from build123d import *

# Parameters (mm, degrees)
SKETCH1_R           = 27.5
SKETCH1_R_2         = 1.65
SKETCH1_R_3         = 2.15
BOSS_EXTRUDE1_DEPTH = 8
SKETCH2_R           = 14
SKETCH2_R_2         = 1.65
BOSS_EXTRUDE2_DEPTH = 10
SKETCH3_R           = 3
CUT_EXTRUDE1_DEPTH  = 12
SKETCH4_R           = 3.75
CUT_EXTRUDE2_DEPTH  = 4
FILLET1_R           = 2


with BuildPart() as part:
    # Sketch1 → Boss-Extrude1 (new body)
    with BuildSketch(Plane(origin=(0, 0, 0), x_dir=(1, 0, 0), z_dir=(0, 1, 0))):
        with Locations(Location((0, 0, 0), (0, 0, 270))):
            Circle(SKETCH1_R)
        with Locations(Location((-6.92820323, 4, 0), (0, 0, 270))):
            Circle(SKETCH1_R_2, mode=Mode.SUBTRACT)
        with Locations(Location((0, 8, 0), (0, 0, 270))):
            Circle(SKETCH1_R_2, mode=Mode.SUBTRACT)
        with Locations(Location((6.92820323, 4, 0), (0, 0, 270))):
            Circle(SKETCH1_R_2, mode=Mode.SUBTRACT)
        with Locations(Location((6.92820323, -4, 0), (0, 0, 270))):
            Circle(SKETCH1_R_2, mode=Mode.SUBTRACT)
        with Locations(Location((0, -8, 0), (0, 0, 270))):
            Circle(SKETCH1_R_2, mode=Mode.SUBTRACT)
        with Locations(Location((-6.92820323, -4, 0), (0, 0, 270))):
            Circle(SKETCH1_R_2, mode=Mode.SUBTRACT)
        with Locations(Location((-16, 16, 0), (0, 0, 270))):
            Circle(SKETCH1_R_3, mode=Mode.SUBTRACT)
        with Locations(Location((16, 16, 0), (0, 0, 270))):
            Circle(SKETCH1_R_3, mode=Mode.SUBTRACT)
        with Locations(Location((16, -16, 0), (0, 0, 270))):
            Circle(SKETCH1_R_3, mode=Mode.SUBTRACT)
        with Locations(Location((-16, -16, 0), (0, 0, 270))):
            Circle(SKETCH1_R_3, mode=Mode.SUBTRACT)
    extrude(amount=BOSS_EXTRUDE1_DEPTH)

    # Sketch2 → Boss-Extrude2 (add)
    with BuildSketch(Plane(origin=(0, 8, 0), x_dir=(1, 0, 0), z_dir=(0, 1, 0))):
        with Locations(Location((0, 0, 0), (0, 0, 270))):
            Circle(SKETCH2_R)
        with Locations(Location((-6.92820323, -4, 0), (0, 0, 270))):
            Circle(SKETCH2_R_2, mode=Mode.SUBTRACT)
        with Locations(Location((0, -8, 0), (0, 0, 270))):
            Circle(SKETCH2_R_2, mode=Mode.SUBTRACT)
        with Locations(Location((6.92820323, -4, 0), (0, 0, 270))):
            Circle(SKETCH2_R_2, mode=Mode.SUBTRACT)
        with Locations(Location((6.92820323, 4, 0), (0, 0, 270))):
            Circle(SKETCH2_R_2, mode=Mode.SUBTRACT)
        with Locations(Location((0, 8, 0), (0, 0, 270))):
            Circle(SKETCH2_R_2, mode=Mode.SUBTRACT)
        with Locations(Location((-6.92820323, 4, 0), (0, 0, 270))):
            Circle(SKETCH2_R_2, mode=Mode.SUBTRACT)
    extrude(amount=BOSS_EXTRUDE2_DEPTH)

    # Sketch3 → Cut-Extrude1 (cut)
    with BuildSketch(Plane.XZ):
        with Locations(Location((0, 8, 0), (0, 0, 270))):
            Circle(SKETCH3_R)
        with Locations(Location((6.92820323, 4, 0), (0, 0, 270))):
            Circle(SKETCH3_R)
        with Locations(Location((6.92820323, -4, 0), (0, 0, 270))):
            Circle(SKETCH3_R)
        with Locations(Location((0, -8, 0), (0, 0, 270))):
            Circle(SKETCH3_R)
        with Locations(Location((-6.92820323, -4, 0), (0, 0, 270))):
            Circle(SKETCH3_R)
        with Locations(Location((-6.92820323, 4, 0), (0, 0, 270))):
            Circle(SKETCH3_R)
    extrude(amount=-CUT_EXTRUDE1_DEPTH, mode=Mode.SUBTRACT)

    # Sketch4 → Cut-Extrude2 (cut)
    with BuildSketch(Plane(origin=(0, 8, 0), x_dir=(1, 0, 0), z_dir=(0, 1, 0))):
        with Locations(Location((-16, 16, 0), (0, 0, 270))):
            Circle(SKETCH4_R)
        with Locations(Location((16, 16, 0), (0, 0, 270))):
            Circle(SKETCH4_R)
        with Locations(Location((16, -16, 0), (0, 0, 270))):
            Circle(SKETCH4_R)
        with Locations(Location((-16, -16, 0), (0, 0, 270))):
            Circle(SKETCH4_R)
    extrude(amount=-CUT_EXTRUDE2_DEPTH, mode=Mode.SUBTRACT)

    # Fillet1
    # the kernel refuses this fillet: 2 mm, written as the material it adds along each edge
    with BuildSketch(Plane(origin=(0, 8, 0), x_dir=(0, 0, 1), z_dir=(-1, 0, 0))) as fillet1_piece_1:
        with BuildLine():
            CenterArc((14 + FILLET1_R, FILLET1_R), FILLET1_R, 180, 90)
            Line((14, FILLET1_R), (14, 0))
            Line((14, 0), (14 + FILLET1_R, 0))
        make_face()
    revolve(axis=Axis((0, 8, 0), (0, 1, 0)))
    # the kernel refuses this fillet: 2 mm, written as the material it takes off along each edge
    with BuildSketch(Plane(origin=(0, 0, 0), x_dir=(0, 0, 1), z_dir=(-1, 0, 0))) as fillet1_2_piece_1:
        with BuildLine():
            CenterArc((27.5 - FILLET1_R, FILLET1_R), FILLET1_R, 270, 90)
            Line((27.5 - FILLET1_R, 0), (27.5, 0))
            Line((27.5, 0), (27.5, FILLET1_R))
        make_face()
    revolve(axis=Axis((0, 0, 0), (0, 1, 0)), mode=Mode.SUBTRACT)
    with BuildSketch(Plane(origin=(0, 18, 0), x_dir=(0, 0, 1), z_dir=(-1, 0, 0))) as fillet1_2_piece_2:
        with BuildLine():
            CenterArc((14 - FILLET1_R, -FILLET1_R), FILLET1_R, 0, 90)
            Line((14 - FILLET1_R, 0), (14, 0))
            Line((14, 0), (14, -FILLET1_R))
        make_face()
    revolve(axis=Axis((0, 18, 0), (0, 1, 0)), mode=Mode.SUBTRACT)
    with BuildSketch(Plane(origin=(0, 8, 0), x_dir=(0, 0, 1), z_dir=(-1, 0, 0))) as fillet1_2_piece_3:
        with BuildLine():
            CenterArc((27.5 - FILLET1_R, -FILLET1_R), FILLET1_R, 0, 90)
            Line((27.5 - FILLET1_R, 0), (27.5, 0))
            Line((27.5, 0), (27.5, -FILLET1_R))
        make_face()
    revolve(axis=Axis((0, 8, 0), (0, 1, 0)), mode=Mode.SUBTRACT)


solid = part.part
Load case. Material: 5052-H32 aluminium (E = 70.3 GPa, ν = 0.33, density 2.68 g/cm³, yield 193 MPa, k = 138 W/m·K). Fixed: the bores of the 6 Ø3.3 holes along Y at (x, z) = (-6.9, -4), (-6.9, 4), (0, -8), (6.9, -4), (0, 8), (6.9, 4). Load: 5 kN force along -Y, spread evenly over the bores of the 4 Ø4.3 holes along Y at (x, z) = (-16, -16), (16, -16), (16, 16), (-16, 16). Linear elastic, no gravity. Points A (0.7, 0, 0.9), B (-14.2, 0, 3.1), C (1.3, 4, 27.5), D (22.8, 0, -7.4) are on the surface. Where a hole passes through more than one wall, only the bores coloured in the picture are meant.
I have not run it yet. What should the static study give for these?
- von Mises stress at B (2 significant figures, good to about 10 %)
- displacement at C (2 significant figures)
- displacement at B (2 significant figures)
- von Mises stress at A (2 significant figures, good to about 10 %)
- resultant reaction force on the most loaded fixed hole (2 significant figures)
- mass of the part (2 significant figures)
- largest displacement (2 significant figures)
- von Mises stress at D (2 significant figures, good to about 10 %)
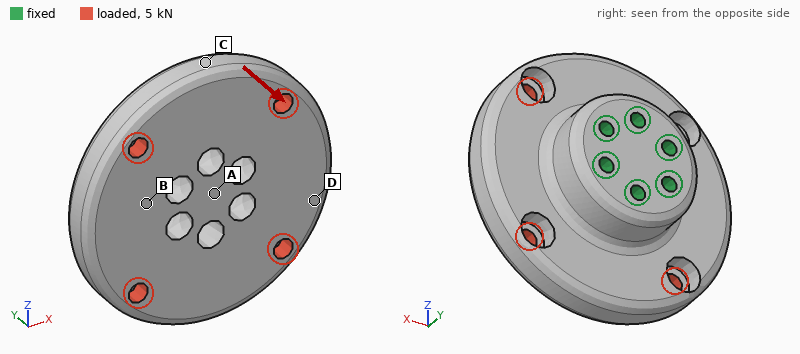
28 MPa
11 µm
5.6 µm
14 MPa
890 N
58 g
24 µm
24 MPa
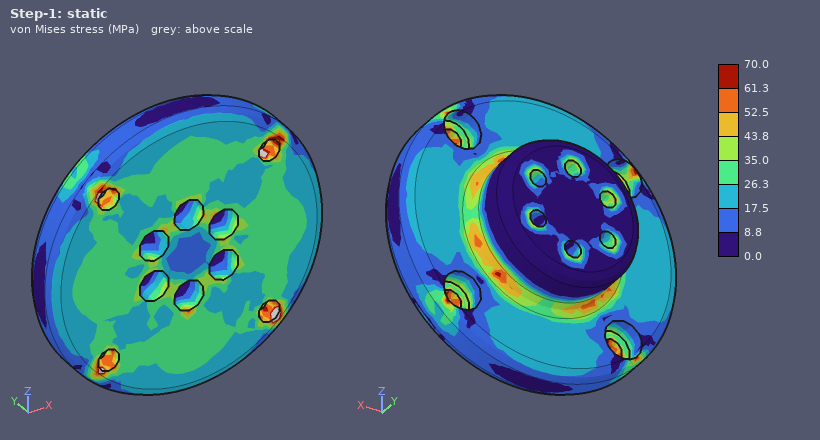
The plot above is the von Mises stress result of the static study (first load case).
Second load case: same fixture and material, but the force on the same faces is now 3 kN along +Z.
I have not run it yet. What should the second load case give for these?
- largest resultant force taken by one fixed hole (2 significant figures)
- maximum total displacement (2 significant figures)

1.2 kN
16 µm
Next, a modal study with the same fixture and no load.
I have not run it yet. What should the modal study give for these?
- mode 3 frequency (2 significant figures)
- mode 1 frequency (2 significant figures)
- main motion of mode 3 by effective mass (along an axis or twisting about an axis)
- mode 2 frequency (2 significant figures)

13 kHz
11 kHz
twisting about Y
11 kHz
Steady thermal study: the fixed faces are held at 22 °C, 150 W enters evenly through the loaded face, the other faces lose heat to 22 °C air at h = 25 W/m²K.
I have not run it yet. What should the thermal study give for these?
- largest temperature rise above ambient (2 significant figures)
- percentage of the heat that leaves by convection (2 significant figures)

56 K
3.6 %
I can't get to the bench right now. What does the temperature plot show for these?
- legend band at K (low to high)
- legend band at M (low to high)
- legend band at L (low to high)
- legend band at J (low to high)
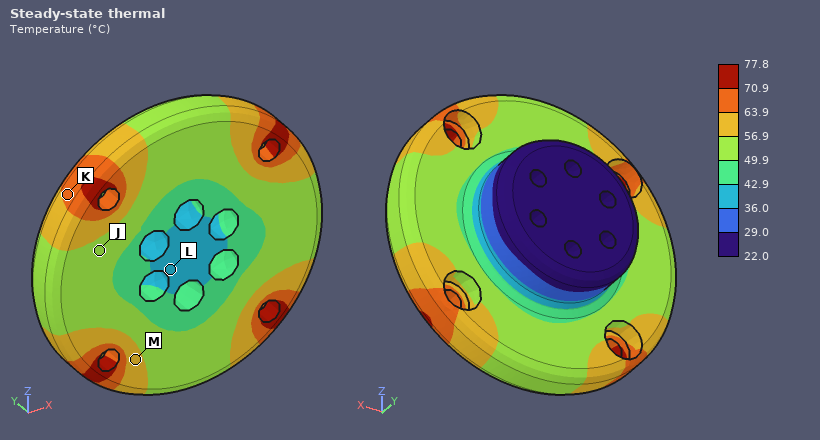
63.9 to 70.9 °C
56.9 to 63.9 °C
36.0 to 42.9 °C
49.9 to 56.9 °C
